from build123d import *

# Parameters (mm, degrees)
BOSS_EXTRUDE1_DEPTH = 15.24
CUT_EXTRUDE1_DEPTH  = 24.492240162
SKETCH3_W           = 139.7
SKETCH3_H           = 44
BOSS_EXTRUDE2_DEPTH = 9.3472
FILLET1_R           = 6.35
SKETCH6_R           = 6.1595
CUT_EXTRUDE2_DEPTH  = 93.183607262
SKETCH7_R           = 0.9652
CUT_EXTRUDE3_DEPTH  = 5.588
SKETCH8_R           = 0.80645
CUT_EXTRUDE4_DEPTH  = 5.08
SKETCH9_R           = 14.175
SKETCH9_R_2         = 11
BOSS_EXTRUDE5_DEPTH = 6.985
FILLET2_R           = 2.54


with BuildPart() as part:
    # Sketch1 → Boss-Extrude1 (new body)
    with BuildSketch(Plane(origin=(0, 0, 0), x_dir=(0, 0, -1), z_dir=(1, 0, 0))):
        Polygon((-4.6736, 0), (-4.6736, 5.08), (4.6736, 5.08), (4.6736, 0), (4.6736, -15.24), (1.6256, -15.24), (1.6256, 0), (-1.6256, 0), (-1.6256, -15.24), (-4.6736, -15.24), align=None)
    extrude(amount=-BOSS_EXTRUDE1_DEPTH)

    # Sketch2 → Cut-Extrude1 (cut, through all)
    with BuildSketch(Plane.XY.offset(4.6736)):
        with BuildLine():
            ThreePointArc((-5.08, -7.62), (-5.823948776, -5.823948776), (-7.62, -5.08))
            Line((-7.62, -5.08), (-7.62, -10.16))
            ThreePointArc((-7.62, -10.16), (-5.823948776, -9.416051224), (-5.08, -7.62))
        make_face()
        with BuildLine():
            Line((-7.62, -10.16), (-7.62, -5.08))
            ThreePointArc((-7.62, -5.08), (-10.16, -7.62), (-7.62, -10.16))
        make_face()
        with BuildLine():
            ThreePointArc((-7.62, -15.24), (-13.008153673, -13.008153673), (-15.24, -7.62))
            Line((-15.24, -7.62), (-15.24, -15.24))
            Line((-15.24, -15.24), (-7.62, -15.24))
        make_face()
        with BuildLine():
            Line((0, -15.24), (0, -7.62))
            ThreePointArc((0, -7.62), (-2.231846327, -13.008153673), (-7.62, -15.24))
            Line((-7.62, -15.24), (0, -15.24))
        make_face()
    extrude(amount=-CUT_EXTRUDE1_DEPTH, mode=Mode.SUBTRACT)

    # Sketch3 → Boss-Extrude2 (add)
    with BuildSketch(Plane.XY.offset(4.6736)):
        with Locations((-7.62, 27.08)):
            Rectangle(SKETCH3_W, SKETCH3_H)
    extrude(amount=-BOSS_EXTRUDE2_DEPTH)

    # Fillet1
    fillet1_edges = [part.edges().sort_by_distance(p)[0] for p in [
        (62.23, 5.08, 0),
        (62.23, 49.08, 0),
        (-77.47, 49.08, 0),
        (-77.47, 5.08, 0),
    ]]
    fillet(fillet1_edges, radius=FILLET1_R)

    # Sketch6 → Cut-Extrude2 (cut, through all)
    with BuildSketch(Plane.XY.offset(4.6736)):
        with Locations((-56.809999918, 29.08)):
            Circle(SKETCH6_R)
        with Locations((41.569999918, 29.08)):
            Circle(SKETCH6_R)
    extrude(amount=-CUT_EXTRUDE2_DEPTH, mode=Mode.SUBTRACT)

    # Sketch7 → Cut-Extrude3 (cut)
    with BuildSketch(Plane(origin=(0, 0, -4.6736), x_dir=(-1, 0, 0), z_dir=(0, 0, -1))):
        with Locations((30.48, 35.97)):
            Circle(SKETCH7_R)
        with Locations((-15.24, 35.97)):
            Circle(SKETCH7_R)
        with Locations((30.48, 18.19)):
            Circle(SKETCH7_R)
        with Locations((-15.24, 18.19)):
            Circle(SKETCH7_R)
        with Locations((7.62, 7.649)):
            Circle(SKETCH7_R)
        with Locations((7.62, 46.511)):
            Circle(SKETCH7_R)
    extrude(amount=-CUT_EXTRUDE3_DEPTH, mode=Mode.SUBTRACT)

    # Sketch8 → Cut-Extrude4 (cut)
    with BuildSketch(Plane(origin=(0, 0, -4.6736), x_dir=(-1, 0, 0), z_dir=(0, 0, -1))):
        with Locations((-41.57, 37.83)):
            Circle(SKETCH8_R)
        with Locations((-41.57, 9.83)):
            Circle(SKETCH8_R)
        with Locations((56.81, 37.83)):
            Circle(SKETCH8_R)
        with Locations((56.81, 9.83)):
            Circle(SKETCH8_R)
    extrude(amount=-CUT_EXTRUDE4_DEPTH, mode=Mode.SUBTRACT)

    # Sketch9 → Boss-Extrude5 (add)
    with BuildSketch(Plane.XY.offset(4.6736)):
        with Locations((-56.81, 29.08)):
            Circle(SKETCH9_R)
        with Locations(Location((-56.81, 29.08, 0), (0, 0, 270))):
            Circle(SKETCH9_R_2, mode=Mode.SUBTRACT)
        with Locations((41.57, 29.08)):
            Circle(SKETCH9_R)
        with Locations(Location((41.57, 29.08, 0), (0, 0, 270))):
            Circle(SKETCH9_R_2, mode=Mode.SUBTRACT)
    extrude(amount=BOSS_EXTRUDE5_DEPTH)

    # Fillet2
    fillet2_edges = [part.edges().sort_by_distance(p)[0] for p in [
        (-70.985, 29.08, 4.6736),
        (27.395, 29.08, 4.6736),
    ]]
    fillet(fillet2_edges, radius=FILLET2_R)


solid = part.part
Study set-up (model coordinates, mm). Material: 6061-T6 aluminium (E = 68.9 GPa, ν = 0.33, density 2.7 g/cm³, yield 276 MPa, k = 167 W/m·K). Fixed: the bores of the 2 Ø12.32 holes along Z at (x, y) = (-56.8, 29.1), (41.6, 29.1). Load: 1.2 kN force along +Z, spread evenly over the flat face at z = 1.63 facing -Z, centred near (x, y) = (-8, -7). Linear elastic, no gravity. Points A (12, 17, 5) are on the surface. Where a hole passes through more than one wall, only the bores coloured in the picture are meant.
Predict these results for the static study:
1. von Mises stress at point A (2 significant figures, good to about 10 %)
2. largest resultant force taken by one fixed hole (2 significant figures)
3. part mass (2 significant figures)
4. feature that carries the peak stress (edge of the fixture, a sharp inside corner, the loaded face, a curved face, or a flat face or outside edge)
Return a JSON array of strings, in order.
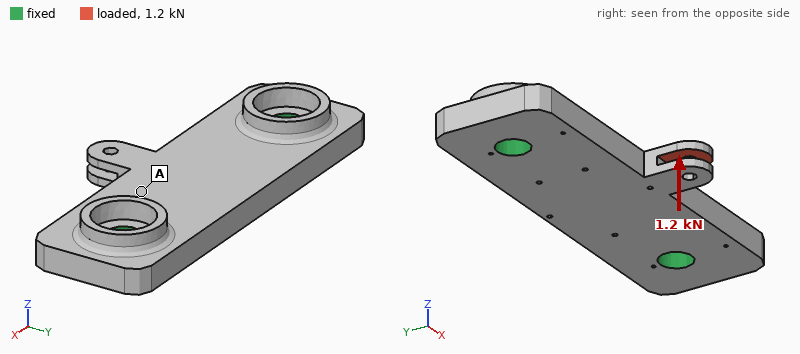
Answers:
["35 MPa", "600 N", "160 g", "a flat face or outside edge"]
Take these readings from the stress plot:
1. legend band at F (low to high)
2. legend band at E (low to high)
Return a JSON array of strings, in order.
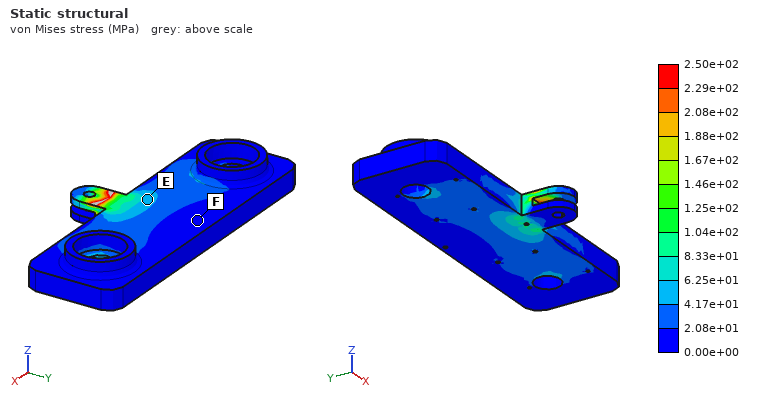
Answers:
["0.00e+00 to 2.08e+01 MPa", "4.17e+01 to 6.25e+01 MPa"]
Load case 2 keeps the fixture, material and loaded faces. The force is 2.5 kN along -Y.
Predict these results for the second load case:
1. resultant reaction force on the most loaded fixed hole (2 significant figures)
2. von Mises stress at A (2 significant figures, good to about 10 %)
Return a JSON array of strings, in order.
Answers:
["1.3 kN", "12 MPa"]
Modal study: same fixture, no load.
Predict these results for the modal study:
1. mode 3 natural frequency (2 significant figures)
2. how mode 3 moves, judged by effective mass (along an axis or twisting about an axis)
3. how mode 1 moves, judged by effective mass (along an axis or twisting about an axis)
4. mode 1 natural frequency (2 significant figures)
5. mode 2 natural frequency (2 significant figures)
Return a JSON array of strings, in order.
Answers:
["10 kHz", "along Y", "along Z", "4400 Hz", "6100 Hz"]
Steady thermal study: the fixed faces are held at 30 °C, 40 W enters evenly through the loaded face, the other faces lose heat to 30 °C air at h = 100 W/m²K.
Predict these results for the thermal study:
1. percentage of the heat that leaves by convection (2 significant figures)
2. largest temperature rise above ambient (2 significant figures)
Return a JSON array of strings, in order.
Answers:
["26 %", "79 K"]
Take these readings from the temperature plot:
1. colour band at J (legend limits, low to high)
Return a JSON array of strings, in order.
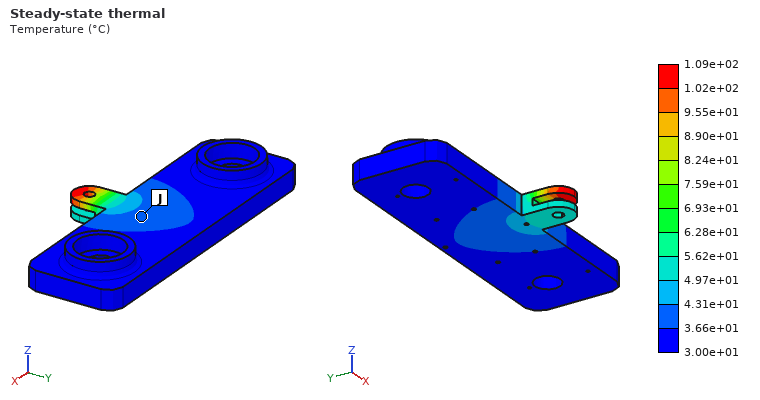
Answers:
["3.66e+01 to 4.31e+01 °C"]
